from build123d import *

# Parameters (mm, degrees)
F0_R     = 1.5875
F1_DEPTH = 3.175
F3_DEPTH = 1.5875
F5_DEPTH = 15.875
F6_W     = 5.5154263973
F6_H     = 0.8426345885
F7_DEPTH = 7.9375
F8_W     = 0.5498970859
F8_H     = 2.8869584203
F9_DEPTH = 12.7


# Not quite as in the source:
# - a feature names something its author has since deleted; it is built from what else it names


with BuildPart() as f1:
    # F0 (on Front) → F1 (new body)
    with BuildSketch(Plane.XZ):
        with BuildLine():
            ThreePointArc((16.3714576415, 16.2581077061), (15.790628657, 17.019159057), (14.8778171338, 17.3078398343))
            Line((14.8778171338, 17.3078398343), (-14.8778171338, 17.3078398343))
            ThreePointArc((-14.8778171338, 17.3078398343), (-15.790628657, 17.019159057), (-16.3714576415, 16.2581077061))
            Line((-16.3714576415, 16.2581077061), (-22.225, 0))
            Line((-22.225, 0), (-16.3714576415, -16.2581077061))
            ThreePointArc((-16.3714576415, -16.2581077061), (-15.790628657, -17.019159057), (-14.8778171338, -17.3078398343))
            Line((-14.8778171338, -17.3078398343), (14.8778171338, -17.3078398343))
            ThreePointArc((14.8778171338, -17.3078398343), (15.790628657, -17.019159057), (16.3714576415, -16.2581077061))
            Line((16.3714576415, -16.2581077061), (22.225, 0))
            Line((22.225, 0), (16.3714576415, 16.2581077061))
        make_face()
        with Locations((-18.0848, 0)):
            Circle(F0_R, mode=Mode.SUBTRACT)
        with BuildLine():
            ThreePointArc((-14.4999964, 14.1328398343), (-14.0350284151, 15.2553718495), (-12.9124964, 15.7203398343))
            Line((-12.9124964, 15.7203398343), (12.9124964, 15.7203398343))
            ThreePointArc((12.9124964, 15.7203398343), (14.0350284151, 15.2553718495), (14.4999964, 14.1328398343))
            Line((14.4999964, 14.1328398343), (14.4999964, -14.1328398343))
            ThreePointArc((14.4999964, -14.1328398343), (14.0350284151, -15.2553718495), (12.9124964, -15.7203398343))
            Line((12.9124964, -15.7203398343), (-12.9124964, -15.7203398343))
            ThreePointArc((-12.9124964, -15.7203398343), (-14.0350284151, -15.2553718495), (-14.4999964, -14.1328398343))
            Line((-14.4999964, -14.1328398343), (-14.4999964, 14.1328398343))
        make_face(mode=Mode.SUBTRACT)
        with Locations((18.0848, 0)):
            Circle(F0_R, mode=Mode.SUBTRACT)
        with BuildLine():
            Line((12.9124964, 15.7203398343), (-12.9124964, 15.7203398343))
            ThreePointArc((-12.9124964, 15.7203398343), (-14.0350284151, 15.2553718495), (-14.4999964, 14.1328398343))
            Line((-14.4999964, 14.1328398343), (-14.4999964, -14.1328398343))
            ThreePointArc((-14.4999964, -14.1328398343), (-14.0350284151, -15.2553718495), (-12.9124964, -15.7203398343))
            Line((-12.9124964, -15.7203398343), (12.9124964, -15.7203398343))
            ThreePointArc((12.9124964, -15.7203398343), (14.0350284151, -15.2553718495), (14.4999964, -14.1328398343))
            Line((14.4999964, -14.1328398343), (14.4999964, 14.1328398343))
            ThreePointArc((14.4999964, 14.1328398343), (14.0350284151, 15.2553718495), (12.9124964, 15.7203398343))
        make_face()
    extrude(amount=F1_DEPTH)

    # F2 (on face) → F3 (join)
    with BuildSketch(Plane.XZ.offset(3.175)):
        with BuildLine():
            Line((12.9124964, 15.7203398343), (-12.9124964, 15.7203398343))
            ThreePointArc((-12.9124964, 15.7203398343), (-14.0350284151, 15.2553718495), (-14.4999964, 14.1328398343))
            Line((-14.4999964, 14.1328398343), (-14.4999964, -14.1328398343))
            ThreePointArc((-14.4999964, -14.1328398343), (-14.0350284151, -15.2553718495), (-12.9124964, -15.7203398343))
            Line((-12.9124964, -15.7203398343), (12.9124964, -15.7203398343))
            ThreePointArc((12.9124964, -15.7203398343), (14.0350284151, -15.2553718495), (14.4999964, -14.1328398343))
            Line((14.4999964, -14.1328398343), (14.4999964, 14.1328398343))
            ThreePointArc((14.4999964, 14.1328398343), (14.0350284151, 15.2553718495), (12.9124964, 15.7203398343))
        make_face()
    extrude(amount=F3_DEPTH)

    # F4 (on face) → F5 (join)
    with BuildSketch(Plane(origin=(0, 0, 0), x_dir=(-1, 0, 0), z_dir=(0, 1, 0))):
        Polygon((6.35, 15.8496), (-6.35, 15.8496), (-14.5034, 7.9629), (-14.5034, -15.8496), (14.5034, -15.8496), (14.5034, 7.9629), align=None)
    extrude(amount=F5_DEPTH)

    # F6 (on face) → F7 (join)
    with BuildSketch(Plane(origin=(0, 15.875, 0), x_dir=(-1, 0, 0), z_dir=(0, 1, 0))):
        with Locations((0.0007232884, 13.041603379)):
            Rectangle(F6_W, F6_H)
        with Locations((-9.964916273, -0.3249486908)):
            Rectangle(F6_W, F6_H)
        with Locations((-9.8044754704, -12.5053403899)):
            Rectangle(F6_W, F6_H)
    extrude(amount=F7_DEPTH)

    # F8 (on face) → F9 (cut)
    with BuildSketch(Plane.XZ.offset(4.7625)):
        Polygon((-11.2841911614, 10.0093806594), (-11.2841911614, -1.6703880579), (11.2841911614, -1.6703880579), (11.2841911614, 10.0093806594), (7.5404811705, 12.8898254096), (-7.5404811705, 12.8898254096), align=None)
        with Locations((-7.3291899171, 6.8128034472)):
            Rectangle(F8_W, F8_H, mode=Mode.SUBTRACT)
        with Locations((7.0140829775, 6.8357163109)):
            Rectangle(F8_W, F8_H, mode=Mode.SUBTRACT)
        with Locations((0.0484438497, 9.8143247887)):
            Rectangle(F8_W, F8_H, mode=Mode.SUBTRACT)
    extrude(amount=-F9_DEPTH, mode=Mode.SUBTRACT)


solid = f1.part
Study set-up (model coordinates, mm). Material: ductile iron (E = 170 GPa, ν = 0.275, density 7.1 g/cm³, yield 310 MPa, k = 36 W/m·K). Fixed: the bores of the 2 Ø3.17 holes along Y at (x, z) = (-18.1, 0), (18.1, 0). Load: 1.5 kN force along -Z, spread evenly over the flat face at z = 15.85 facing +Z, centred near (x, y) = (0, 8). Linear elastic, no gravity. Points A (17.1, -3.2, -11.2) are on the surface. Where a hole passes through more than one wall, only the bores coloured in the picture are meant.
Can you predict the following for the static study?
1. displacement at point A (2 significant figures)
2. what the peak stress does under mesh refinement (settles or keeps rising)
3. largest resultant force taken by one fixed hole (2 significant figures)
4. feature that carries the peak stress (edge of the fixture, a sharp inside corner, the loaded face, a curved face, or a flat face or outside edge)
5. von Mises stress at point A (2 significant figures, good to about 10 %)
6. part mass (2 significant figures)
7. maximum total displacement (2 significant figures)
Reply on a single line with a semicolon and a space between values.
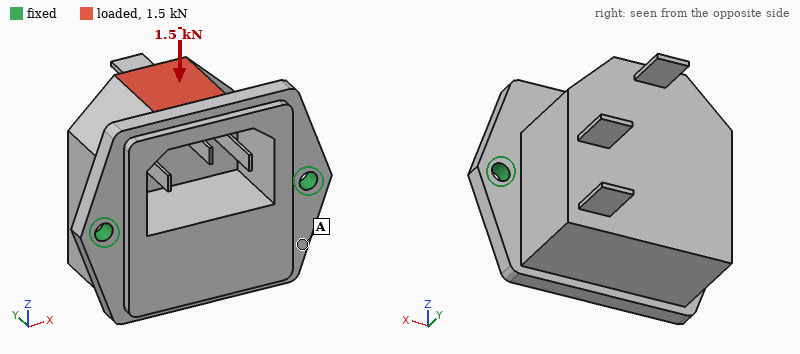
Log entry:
26 µm; keeps rising; 750 N; edge of the fixture; 34 MPa; 110 g; 73 µm
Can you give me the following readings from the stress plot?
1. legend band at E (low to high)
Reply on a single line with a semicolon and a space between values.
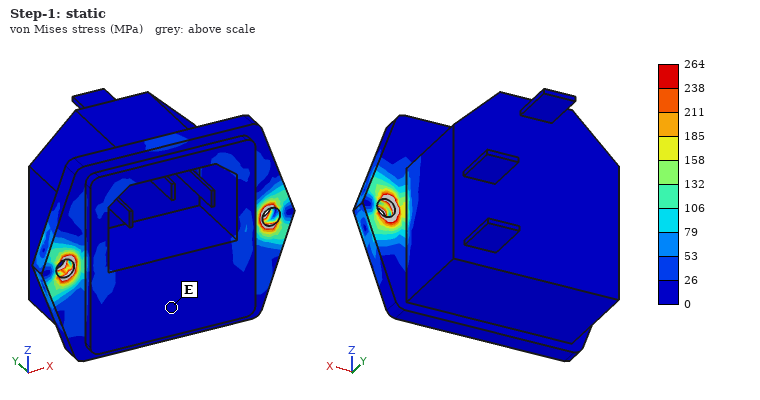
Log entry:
0 to 26 MPa
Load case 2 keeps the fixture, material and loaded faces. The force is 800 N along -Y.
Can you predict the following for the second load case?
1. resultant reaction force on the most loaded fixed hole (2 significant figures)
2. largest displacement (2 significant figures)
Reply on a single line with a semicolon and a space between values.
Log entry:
480 N; 69 µm
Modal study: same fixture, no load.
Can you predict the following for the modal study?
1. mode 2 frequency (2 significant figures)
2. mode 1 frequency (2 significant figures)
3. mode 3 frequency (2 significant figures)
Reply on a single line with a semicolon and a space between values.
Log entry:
2700 Hz; 2700 Hz; 2700 Hz
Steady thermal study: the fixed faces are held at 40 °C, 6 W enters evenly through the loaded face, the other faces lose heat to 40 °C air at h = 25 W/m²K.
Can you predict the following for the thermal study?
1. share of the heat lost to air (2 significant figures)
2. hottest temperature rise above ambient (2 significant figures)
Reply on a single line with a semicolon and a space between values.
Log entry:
26 %; 22 K
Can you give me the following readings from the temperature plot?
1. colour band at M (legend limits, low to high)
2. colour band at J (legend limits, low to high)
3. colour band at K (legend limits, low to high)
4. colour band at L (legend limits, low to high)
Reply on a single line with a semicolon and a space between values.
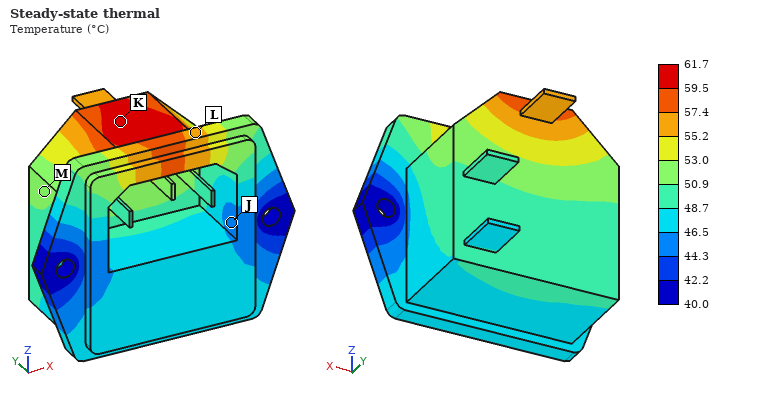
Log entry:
50.9 to 53.0 °C; 44.3 to 46.5 °C; 59.5 to 61.7 °C; 55.2 to 57.4 °C
